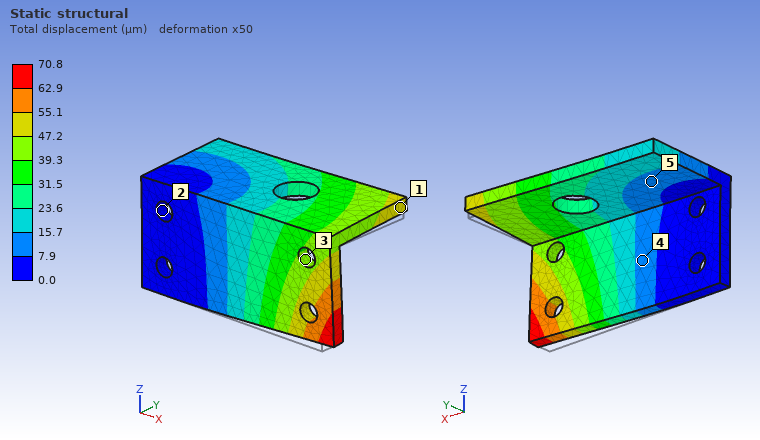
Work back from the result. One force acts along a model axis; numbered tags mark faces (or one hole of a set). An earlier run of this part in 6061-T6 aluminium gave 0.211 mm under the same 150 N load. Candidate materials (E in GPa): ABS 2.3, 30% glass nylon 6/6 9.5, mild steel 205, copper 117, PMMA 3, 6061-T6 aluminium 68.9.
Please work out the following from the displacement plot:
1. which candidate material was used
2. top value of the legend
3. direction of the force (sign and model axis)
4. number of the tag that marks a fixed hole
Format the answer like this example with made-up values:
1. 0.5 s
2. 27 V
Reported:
1. mild steel
2. 70.8 µm
3. +Y
4. 2
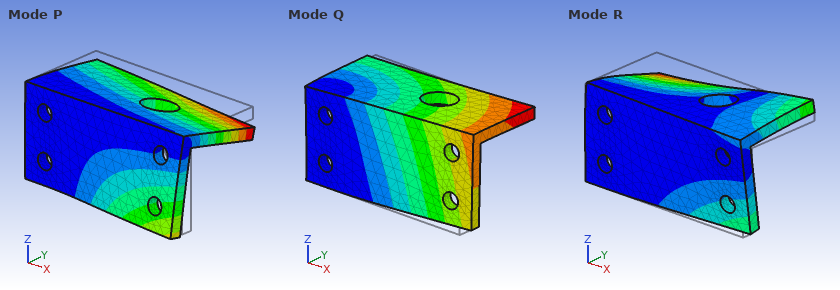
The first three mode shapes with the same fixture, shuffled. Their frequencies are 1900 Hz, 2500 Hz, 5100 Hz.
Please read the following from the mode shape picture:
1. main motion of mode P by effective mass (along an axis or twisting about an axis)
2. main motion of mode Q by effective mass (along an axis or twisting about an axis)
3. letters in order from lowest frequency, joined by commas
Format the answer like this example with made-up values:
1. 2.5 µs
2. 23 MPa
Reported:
1. along Z
2. along Y
3. Q, P, R
